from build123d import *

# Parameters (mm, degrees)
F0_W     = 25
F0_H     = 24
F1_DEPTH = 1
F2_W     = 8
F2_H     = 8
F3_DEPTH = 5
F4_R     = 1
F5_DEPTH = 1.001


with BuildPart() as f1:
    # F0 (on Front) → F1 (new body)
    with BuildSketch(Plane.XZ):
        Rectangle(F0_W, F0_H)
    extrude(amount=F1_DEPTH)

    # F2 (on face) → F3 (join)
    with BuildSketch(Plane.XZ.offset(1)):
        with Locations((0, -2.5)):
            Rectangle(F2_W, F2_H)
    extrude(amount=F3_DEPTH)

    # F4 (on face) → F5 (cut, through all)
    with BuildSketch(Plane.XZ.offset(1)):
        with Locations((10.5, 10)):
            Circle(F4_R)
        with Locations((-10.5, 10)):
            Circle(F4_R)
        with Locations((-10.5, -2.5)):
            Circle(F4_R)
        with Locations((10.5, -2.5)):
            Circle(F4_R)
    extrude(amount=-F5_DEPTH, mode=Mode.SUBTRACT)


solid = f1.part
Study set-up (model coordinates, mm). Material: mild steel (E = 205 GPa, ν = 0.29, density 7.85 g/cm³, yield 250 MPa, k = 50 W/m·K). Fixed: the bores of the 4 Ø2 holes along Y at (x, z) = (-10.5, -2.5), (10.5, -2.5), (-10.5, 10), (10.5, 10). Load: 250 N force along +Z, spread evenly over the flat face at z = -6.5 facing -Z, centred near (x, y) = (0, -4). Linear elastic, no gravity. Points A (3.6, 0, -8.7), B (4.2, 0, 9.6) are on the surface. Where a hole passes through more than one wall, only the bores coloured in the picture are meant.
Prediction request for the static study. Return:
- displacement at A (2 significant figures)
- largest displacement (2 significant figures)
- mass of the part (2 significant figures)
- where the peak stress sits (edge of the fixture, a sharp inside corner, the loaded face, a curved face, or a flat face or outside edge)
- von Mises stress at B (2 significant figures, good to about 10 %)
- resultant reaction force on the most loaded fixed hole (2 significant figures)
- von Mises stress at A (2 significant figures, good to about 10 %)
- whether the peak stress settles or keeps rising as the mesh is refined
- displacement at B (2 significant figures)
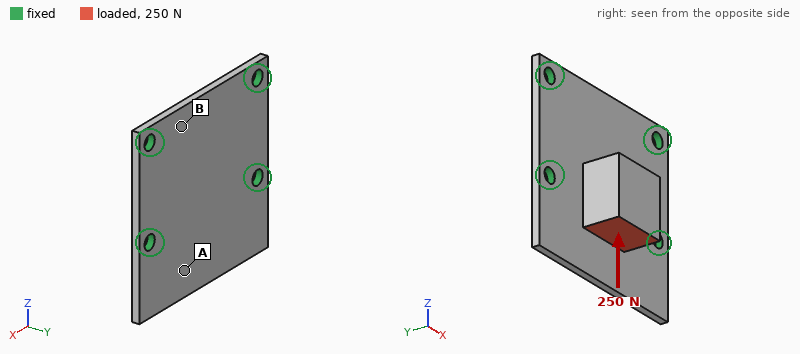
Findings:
20 µm
30 µm
7.1 g
edge of the fixture
19 MPa
81 N
42 MPa
keeps rising
5.8 µm
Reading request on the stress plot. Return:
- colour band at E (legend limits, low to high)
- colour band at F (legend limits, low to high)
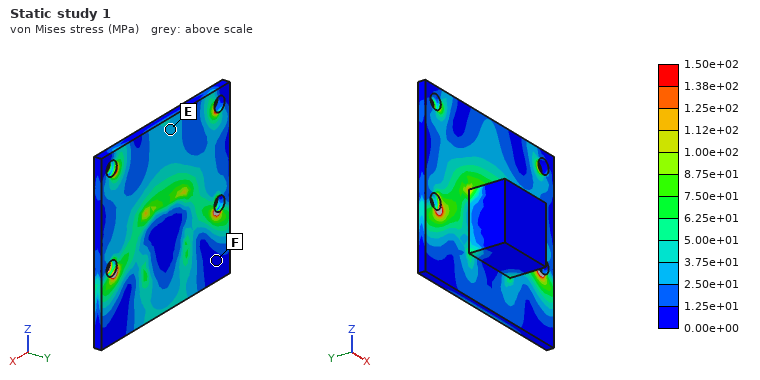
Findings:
2.50e+01 to 3.75e+01 MPa
0.00e+00 to 1.25e+01 MPa
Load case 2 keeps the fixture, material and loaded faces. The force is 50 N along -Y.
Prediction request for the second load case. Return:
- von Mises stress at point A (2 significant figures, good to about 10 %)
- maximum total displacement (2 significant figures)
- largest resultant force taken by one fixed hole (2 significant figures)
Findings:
23 MPa
14 µm
32 N
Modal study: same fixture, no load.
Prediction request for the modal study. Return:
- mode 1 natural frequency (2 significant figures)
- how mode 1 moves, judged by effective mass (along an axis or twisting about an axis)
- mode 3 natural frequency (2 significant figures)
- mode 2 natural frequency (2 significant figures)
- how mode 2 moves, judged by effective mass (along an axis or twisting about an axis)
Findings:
7200 Hz
along Y
14 kHz
10 kHz
along Y
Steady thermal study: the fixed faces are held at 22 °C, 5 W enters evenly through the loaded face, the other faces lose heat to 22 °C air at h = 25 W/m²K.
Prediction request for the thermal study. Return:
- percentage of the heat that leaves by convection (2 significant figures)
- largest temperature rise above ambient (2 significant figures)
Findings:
9.6 %
35 K
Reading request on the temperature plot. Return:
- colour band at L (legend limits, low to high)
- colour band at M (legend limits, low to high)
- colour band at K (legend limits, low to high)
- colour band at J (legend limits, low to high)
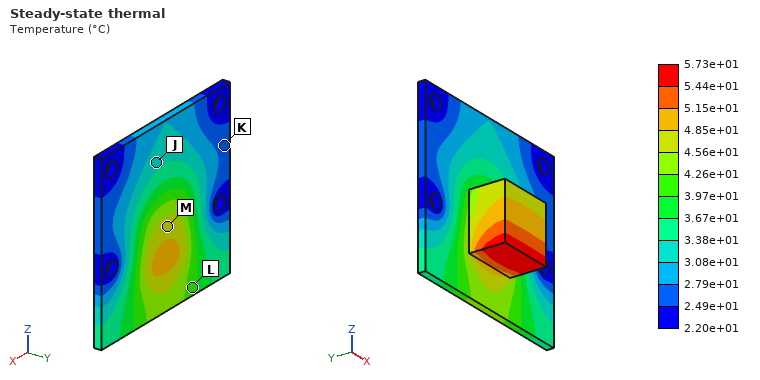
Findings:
3.97e+01 to 4.26e+01 °C
4.56e+01 to 4.85e+01 °C
2.49e+01 to 2.79e+01 °C
3.08e+01 to 3.38e+01 °C
